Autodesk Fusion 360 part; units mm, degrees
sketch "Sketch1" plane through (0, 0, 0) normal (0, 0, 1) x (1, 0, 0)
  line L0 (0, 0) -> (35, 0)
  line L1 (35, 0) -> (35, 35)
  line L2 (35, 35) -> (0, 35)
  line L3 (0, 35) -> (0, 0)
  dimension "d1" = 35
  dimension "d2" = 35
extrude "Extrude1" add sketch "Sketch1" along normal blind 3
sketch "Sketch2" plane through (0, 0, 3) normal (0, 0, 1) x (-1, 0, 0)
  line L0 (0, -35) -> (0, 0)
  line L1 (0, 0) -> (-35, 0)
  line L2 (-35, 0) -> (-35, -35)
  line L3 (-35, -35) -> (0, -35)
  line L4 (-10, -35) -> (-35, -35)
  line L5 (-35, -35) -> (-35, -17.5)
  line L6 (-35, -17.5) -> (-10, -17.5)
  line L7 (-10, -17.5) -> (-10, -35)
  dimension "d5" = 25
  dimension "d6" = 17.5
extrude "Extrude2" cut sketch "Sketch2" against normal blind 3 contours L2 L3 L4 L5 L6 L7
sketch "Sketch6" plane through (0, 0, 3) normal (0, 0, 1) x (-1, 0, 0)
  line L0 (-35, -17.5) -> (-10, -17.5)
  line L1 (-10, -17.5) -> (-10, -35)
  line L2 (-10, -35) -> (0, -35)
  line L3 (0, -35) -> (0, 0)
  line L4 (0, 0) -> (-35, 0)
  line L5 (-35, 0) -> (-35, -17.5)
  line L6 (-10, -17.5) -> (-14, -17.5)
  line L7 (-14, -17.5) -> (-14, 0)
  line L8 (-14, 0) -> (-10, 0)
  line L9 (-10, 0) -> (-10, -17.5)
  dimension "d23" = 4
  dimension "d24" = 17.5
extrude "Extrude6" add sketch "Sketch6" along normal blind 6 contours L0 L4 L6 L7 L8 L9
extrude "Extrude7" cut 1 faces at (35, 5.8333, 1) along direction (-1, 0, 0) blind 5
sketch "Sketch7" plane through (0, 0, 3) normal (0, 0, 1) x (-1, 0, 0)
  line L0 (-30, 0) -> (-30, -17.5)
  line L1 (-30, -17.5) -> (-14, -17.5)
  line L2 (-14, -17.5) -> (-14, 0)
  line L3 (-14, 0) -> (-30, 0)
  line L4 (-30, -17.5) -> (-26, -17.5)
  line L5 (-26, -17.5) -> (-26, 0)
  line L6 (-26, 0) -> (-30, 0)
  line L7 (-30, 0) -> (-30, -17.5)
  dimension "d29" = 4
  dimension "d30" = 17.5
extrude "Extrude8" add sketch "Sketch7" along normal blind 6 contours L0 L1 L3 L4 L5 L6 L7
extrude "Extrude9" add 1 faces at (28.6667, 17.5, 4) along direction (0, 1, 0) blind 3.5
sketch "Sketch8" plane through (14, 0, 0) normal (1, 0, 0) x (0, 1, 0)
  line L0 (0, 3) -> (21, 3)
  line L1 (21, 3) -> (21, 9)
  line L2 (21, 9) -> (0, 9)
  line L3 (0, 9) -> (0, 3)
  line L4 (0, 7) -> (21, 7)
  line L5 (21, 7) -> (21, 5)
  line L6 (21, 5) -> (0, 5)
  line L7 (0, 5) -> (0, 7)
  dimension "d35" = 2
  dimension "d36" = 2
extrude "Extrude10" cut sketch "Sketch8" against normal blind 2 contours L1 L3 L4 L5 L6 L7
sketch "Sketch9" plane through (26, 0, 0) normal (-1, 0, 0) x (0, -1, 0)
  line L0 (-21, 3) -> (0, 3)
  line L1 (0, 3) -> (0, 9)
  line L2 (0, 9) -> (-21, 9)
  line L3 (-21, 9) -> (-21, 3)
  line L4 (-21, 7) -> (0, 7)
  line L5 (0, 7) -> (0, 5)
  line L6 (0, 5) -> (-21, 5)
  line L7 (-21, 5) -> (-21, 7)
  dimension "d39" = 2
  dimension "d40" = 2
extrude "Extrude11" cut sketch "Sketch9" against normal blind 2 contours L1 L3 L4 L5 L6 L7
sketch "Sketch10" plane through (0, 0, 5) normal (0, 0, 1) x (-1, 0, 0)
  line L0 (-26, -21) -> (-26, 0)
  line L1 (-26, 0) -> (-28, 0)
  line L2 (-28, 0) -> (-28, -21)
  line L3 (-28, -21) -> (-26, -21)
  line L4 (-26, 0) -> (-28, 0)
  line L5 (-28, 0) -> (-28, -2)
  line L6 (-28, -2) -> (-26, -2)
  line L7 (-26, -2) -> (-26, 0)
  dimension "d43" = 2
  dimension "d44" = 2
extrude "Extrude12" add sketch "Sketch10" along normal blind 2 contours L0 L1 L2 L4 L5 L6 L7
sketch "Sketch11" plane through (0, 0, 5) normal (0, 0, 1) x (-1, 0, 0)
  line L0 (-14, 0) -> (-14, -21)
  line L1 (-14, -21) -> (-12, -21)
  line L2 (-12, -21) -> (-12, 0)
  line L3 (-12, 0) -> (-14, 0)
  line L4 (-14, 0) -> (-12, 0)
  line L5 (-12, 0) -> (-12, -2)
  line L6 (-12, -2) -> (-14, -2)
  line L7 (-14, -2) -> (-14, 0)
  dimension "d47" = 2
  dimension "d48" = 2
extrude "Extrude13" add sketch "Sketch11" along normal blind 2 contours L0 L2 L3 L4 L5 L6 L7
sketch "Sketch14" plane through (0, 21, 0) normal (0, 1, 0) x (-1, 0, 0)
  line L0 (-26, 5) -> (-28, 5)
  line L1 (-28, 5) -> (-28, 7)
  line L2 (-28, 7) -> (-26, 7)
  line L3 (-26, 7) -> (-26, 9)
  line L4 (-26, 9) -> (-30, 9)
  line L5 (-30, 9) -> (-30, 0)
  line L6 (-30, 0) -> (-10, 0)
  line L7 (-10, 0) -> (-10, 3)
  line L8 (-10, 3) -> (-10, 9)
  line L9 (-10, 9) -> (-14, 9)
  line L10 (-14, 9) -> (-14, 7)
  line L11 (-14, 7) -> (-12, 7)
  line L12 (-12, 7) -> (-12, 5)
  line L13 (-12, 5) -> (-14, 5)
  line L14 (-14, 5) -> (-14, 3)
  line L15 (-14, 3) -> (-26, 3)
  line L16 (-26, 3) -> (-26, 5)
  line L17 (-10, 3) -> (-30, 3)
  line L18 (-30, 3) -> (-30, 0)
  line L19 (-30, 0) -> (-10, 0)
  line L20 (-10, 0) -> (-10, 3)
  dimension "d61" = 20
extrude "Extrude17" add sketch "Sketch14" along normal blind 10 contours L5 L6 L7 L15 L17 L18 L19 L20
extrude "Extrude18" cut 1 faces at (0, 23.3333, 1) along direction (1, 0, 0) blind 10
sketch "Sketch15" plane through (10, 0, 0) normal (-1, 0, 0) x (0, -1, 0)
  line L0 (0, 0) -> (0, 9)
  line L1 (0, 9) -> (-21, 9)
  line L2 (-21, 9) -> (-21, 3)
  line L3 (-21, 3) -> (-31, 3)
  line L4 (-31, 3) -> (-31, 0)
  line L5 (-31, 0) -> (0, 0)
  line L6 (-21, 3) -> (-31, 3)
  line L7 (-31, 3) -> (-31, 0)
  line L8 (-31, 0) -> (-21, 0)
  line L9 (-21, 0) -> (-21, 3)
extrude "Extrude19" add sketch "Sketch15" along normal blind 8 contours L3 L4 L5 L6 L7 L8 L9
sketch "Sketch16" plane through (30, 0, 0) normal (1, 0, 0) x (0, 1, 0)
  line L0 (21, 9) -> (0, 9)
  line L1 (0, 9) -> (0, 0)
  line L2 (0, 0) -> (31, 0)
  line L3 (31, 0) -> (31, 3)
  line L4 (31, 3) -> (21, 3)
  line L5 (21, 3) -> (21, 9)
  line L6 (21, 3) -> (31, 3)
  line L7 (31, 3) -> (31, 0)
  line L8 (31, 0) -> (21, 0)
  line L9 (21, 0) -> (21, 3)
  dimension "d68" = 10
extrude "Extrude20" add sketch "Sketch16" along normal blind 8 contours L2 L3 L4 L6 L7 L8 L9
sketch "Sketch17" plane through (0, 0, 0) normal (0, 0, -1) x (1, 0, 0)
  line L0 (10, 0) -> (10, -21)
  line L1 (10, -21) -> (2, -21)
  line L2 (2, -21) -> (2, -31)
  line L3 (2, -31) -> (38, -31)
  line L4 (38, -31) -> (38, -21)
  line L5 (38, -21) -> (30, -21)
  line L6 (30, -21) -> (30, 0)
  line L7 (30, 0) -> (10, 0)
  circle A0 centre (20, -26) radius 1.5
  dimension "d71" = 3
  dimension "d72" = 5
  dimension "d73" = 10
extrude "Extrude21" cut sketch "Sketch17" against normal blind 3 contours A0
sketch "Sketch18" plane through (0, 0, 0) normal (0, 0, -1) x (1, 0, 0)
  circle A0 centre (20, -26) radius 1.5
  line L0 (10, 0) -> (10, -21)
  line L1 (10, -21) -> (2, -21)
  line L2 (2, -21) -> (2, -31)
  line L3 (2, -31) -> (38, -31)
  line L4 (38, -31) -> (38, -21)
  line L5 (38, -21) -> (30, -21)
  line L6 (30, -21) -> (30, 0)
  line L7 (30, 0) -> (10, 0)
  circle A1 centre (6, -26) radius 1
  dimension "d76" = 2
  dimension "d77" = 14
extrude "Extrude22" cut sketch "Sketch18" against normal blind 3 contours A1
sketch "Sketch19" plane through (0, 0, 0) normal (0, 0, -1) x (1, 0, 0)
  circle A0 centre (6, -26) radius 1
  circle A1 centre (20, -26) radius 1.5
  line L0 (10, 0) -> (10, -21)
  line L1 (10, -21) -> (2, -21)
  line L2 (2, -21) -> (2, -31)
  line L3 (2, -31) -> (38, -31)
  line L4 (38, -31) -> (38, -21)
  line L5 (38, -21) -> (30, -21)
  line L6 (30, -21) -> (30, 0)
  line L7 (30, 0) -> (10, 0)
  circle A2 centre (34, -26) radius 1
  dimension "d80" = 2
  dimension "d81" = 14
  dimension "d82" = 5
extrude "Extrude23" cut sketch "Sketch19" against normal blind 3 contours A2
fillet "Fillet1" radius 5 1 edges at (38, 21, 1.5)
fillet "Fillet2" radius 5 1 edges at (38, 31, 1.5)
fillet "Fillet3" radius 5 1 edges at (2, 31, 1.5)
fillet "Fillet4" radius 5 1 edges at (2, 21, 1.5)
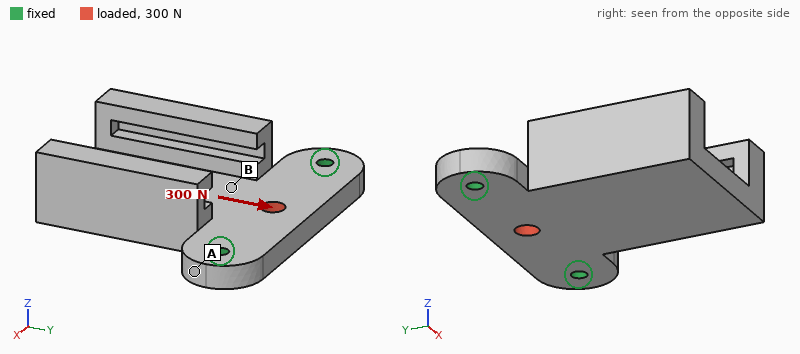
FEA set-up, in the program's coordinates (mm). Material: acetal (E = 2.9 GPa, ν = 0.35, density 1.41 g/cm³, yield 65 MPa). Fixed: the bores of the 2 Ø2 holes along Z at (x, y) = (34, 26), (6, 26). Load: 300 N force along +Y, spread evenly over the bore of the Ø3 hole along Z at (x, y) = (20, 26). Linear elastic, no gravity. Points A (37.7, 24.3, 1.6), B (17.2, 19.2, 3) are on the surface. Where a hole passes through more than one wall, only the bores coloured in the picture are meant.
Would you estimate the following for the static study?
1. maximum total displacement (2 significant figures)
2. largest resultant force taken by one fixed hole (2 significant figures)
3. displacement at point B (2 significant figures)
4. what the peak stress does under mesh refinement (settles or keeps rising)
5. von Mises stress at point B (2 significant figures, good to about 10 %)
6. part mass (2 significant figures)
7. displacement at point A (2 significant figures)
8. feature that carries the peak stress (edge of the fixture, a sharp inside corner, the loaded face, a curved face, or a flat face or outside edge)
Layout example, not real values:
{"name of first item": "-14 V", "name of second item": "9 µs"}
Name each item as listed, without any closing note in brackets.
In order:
{"maximum total displacement": "0.11 mm", "largest resultant force taken by one fixed hole": "160 N", "displacement at point B": "0.074 mm", "what the peak stress does under mesh refinement": "keeps rising", "von Mises stress at point B": "8.7 MPa", "part mass": "4.4 g", "displacement at point A": "0.016 mm", "feature that carries the peak stress": "edge of the fixture"}
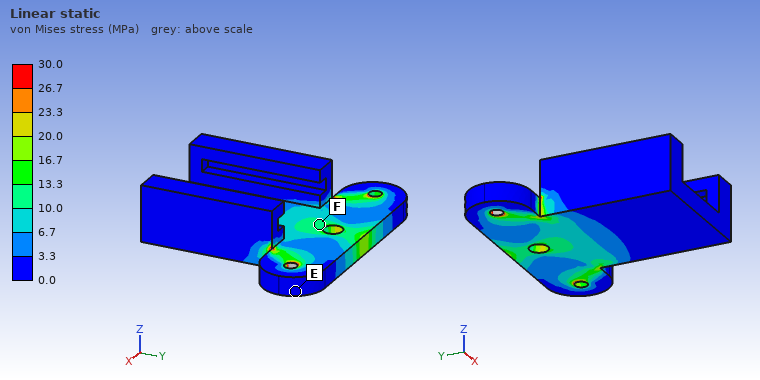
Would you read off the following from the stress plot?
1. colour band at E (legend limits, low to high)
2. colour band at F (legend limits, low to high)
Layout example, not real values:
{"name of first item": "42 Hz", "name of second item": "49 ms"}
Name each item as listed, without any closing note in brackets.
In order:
{"colour band at E": "0.0 to 3.3 MPa", "colour band at F": "10.0 to 13.3 MPa"}
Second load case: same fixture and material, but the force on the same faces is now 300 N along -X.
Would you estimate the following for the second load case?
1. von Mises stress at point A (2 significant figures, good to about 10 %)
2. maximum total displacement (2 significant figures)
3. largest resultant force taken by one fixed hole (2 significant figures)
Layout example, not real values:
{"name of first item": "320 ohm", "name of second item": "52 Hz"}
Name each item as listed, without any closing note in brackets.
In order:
{"von Mises stress at point A": "3.0 MPa", "maximum total displacement": "33 µm", "largest resultant force taken by one fixed hole": "150 N"}
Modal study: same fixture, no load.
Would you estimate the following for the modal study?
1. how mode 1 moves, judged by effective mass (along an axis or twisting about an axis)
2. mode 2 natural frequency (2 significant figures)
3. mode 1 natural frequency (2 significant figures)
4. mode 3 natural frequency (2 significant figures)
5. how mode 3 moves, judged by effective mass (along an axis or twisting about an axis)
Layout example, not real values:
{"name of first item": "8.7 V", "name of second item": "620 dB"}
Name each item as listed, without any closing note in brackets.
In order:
{"how mode 1 moves, judged by effective mass": "along Z", "mode 2 natural frequency": "2100 Hz", "mode 1 natural frequency": "660 Hz", "mode 3 natural frequency": "3800 Hz", "how mode 3 moves, judged by effective mass": "along X"}
